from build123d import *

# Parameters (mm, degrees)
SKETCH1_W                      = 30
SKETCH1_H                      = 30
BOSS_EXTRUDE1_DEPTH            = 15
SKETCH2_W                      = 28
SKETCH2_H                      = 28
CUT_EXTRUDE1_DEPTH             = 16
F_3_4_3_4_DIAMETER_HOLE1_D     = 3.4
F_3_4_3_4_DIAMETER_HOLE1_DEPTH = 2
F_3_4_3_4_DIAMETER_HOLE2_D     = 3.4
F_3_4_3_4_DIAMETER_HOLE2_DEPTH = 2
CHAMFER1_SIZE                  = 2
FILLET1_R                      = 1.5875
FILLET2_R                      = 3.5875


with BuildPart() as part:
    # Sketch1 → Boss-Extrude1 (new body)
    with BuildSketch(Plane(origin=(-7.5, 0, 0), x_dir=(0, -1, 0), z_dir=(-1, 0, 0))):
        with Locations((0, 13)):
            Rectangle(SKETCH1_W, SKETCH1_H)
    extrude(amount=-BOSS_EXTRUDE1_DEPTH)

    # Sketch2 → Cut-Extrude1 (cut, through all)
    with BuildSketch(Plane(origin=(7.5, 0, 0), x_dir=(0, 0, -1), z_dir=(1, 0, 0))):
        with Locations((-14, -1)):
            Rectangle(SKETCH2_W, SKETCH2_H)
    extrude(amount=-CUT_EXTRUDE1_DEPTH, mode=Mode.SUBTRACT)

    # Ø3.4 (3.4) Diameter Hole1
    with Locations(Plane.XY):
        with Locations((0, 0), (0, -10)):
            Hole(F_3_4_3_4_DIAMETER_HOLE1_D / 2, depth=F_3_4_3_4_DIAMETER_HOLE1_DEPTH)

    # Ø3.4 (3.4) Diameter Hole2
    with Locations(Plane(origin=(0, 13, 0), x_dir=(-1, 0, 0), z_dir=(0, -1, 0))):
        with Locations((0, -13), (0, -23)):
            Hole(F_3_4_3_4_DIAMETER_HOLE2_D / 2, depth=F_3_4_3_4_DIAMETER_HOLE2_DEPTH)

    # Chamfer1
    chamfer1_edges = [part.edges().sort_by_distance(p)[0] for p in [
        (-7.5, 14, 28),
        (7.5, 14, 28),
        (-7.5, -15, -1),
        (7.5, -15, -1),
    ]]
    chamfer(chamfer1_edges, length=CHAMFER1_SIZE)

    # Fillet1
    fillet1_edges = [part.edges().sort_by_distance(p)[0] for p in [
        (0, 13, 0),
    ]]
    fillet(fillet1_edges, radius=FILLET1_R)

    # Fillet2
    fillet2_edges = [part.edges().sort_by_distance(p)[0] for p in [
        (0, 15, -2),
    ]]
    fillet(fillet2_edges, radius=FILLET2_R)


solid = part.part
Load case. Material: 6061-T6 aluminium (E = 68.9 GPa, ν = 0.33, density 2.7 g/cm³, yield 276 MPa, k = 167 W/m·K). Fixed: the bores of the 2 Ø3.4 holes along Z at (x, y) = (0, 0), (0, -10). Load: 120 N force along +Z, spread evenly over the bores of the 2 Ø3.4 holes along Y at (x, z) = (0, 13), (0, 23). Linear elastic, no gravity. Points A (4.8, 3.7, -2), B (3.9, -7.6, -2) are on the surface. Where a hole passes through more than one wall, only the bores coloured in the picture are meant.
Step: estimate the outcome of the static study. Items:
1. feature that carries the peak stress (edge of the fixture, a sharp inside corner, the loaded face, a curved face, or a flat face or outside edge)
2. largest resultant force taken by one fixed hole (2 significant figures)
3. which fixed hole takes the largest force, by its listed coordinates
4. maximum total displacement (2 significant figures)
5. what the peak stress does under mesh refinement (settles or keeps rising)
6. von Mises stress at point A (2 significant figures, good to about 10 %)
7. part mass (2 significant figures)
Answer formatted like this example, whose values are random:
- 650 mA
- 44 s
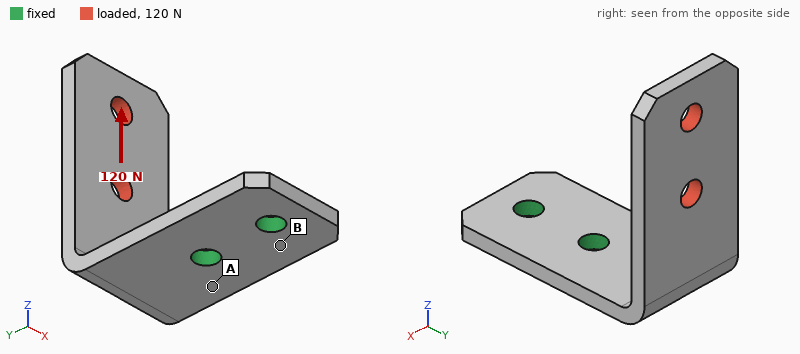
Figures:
- edge of the fixture
- 150 N
- (0, 0)
- 0.47 mm
- keeps rising
- 100 MPa
- 4.4 g
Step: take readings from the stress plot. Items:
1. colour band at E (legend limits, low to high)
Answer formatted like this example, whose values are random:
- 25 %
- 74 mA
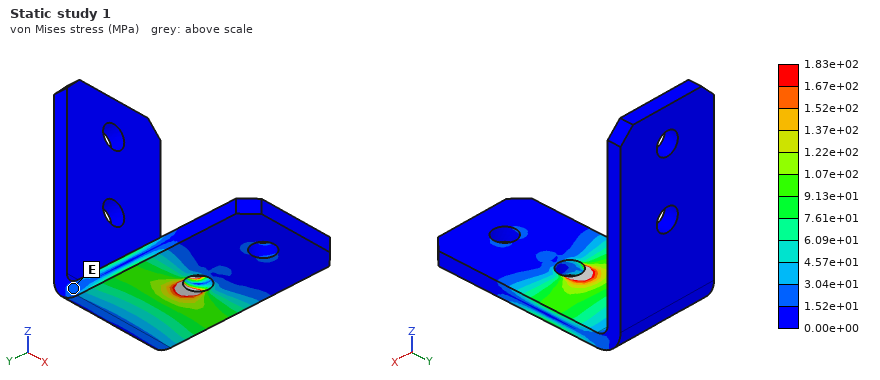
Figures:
- 1.52e+01 to 3.04e+01 MPa
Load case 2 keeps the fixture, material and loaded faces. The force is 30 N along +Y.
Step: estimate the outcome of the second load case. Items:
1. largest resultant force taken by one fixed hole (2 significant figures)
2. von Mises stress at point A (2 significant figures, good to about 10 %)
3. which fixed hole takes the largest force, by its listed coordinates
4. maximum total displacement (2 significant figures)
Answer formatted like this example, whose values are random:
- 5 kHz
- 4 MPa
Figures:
- 28 N
- 49 MPa
- (0, 0)
- 0.47 mm
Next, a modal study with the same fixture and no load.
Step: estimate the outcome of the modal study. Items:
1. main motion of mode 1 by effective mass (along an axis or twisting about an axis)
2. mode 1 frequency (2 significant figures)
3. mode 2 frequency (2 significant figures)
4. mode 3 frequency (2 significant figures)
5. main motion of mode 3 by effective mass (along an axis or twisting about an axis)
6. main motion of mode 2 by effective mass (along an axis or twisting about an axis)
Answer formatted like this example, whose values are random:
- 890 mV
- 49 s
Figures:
- along Y
- 1200 Hz
- 1800 Hz
- 4300 Hz
- along Z
- along X
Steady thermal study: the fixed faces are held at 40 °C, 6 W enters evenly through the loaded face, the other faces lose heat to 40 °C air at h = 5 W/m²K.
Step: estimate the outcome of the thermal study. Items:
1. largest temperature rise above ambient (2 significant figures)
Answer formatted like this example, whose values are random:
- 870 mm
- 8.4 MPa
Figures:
- 40 K
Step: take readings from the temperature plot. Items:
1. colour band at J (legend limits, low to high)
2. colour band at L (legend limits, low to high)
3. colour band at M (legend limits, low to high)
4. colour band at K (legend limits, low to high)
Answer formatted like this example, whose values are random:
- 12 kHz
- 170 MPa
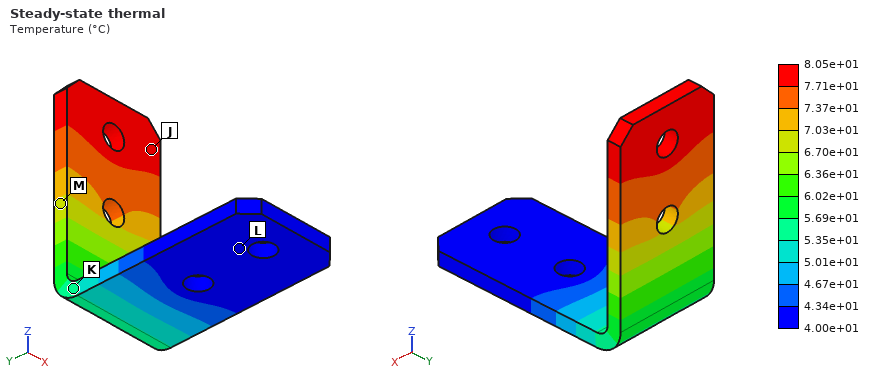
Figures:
- 7.71e+01 to 8.05e+01 °C
- 4.00e+01 to 4.34e+01 °C
- 6.70e+01 to 7.03e+01 °C
- 5.35e+01 to 5.69e+01 °C
